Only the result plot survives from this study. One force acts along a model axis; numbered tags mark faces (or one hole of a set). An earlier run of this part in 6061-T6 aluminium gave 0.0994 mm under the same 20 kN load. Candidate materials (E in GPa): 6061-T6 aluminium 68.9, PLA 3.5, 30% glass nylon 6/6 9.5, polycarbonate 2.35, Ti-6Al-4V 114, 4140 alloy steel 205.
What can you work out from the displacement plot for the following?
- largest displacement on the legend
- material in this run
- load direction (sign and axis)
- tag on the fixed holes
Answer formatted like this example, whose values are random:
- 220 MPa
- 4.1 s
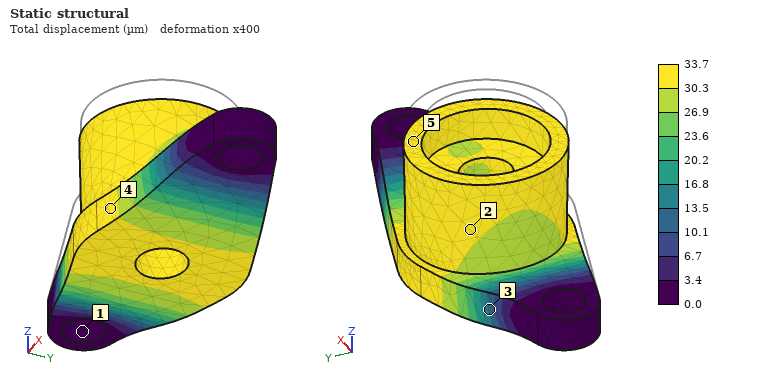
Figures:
- 33.7 µm
- 4140 alloy steel
- -Z
- 1
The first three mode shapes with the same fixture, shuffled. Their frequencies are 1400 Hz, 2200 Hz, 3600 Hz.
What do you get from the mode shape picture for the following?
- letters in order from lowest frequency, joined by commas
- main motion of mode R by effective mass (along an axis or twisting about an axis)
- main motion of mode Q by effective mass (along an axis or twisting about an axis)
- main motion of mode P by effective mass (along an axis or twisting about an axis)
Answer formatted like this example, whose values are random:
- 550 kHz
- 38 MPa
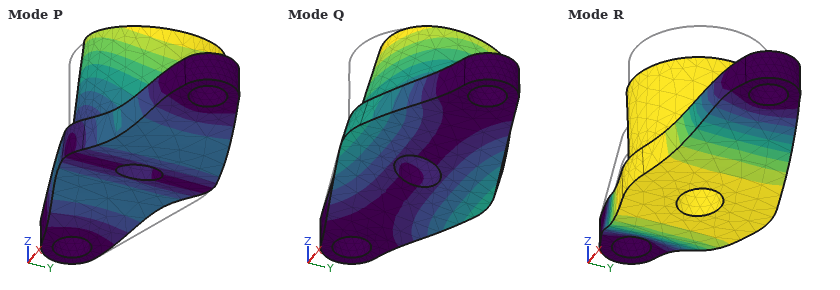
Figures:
- Q, R, P
- along Z
- along Y
- along X
